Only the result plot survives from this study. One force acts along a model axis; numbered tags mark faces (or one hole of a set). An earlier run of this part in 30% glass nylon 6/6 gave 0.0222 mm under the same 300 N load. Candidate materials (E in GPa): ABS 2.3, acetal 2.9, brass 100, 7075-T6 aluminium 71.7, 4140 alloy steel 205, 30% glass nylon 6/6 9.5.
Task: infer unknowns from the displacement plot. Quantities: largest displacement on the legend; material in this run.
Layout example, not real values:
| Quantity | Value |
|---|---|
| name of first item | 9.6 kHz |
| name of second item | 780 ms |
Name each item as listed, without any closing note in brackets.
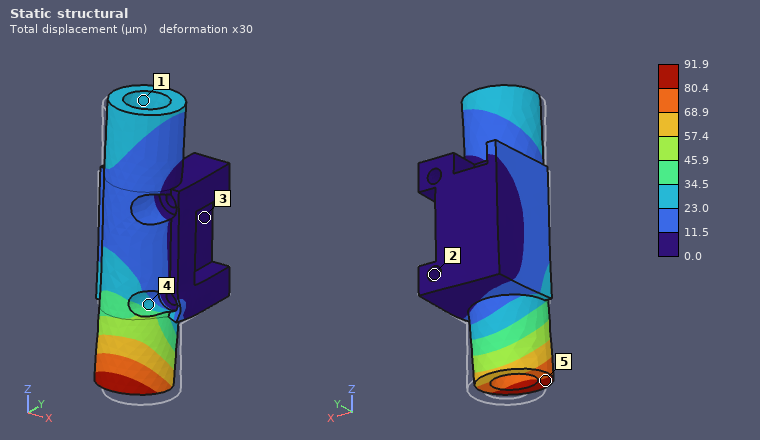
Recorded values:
| Quantity | Value |
|---|---|
| largest displacement on the legend | 91.9 µm |
| material in this run | ABS |
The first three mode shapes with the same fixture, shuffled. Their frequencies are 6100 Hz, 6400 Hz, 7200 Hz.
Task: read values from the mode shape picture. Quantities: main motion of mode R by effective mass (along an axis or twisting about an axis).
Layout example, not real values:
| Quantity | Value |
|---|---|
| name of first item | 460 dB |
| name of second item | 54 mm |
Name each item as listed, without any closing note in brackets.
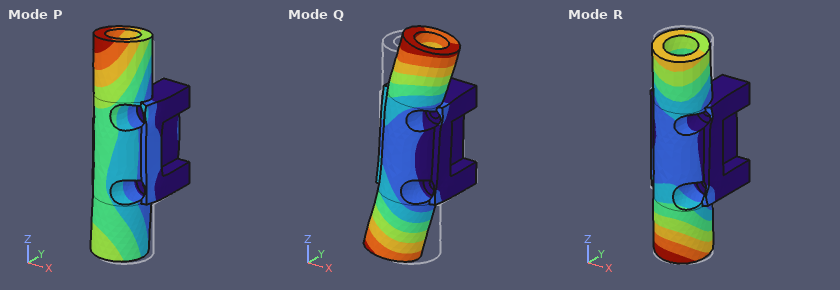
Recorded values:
| Quantity | Value |
|---|---|
| main motion of mode R by effective mass | twisting about X |
